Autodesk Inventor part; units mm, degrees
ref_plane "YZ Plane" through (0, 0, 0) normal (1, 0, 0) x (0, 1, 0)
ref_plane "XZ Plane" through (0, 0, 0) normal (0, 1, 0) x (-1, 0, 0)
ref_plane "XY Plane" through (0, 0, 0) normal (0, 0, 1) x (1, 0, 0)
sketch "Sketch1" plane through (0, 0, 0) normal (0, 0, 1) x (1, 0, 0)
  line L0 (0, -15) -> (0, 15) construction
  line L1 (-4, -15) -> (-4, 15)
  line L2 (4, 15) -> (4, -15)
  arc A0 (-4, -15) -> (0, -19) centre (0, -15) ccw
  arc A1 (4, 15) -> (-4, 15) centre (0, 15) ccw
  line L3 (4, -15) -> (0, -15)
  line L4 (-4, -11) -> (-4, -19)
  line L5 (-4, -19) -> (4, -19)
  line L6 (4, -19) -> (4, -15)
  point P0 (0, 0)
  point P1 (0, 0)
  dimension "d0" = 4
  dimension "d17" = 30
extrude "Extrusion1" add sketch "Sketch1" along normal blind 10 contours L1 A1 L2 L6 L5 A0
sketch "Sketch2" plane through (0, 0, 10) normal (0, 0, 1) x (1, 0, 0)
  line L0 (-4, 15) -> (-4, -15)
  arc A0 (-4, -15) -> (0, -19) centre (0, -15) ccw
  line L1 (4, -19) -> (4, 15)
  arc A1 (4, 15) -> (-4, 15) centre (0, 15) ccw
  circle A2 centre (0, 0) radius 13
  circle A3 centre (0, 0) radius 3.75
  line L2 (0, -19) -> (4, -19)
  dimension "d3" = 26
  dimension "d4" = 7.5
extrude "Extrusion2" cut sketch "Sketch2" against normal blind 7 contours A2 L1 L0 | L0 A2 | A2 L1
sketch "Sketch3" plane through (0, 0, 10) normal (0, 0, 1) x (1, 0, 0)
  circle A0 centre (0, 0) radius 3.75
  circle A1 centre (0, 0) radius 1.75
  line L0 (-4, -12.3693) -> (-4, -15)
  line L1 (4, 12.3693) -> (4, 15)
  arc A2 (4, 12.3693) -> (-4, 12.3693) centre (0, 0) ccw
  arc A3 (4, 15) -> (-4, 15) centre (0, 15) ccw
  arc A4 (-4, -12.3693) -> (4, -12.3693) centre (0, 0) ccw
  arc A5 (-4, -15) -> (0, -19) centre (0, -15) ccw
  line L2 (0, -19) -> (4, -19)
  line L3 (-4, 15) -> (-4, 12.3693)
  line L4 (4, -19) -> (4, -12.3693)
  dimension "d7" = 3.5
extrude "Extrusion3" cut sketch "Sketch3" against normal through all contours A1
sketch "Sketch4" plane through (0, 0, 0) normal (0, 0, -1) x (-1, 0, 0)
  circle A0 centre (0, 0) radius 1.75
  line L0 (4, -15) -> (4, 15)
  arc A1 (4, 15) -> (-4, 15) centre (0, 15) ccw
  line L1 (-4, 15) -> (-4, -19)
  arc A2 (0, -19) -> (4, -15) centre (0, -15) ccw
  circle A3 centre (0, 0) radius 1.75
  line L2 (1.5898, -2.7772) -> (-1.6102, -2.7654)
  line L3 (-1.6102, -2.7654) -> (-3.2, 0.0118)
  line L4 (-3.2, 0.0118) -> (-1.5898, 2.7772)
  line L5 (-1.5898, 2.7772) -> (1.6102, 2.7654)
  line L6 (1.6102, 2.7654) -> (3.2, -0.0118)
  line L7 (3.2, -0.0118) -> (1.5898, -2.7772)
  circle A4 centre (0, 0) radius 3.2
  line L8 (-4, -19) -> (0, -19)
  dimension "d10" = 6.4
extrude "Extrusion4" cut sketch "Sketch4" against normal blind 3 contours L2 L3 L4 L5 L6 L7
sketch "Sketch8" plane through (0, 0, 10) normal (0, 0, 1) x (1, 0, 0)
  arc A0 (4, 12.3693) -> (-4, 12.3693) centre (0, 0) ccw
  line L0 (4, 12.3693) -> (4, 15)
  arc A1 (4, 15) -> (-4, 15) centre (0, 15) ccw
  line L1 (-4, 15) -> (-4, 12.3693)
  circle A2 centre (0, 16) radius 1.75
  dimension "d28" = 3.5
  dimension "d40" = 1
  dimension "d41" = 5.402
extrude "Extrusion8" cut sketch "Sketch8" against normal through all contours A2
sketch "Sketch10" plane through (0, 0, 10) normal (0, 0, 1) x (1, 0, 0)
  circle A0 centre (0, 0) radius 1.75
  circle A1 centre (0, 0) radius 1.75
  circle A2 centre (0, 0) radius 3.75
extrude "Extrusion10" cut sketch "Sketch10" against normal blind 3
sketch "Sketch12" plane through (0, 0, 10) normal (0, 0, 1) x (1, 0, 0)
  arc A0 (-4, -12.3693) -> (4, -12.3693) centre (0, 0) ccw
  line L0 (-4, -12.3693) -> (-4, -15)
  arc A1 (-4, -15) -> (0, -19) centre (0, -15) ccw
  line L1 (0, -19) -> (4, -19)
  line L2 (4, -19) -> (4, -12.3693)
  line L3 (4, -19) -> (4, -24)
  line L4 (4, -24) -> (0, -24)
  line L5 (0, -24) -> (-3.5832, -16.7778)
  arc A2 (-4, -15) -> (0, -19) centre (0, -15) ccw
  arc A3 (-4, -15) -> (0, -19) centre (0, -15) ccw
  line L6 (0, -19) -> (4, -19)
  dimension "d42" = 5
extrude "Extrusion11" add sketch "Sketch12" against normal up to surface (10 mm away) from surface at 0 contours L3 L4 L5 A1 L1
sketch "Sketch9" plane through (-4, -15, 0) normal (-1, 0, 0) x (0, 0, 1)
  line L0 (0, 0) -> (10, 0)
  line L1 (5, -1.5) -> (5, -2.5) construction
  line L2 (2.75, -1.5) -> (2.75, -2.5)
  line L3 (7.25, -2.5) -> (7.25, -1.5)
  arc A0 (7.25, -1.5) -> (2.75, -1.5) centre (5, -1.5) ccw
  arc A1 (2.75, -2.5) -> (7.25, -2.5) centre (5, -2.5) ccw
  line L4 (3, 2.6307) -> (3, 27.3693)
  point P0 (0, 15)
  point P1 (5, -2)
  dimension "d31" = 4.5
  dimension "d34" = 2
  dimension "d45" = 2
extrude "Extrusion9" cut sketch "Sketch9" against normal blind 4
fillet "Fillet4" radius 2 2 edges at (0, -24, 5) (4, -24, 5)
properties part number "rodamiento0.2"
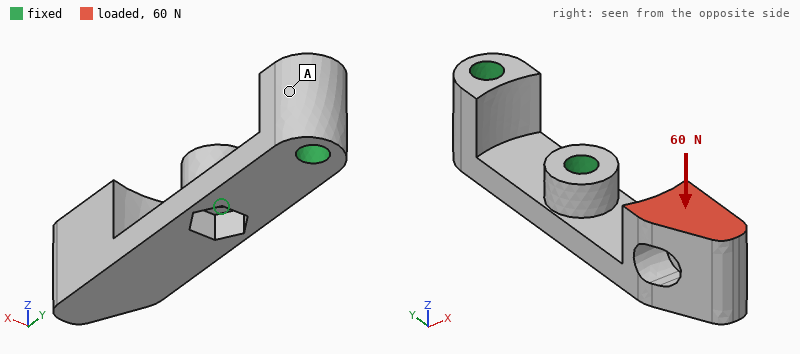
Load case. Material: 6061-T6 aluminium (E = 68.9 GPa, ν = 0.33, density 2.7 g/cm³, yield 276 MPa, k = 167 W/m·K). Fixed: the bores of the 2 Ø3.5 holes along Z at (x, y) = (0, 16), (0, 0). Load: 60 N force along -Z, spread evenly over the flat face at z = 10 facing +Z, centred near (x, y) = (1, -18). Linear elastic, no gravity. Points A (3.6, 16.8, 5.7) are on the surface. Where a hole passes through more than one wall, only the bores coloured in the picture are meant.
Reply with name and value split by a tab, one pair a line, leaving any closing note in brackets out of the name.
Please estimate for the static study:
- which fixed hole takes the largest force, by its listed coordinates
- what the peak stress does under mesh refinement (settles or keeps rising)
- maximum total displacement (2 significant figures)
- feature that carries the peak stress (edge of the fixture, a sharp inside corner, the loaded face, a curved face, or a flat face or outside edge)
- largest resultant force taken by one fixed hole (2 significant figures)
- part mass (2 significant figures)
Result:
which fixed hole takes the largest force, by its listed coordinates	(0, 0)
what the peak stress does under mesh refinement	keeps rising
maximum total displacement	0.15 mm
feature that carries the peak stress	a sharp inside corner
largest resultant force taken by one fixed hole	120 N
part mass	4.5 g
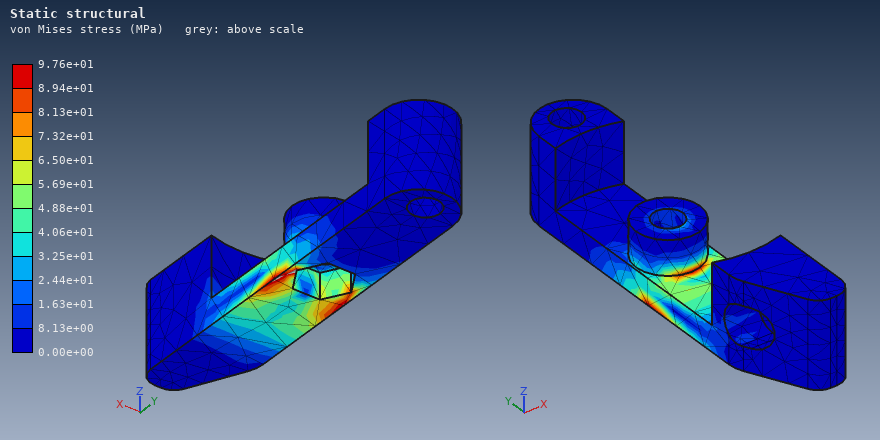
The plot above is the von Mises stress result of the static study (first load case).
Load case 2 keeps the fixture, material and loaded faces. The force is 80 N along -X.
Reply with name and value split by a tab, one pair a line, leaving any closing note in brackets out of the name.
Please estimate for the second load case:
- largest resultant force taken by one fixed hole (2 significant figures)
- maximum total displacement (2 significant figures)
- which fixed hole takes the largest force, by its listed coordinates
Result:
largest resultant force taken by one fixed hole	130 N
maximum total displacement	98 µm
which fixed hole takes the largest force, by its listed coordinates	(0, 0)
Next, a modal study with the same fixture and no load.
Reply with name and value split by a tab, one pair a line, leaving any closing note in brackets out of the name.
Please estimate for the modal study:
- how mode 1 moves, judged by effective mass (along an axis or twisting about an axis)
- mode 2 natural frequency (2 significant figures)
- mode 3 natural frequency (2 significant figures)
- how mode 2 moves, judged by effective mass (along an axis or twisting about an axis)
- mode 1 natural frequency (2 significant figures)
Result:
how mode 1 moves, judged by effective mass	along Z
mode 2 natural frequency	5100 Hz
mode 3 natural frequency	12 kHz
how mode 2 moves, judged by effective mass	along X
mode 1 natural frequency	2800 Hz
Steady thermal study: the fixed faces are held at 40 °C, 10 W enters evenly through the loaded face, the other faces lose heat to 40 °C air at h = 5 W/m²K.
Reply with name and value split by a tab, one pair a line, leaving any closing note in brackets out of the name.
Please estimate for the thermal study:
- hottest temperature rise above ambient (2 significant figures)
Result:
hottest temperature rise above ambient	49 K
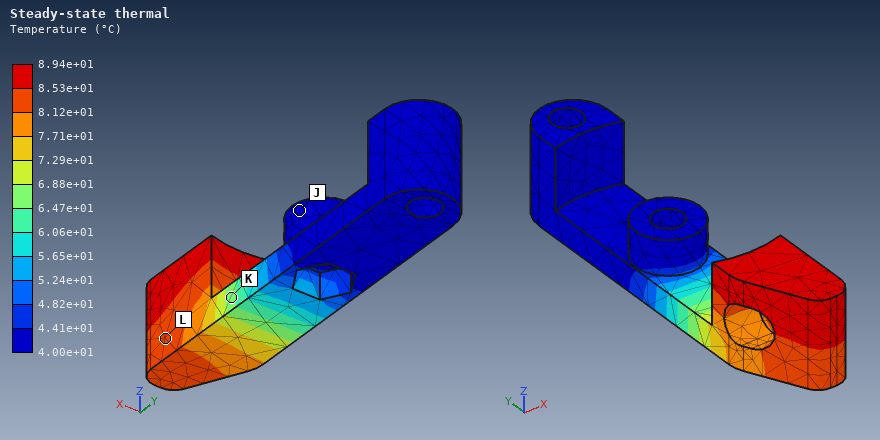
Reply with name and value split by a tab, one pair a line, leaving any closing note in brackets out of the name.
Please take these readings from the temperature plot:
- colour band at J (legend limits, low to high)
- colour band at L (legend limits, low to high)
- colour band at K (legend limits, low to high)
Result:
colour band at J	4.00e+01 to 4.41e+01 °C
colour band at L	8.12e+01 to 8.53e+01 °C
colour band at K	6.47e+01 to 6.88e+01 °C
